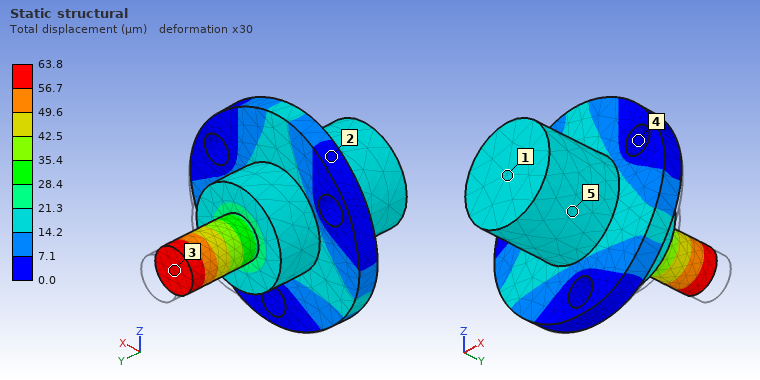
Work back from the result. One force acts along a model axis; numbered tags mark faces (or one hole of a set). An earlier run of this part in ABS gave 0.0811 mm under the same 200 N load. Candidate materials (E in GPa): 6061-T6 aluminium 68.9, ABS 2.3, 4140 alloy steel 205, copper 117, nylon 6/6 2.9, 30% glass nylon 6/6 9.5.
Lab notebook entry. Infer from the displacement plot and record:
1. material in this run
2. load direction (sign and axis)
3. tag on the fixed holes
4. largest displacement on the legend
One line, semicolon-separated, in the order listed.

nylon 6/6; -Y; 4; 63.8 µm
